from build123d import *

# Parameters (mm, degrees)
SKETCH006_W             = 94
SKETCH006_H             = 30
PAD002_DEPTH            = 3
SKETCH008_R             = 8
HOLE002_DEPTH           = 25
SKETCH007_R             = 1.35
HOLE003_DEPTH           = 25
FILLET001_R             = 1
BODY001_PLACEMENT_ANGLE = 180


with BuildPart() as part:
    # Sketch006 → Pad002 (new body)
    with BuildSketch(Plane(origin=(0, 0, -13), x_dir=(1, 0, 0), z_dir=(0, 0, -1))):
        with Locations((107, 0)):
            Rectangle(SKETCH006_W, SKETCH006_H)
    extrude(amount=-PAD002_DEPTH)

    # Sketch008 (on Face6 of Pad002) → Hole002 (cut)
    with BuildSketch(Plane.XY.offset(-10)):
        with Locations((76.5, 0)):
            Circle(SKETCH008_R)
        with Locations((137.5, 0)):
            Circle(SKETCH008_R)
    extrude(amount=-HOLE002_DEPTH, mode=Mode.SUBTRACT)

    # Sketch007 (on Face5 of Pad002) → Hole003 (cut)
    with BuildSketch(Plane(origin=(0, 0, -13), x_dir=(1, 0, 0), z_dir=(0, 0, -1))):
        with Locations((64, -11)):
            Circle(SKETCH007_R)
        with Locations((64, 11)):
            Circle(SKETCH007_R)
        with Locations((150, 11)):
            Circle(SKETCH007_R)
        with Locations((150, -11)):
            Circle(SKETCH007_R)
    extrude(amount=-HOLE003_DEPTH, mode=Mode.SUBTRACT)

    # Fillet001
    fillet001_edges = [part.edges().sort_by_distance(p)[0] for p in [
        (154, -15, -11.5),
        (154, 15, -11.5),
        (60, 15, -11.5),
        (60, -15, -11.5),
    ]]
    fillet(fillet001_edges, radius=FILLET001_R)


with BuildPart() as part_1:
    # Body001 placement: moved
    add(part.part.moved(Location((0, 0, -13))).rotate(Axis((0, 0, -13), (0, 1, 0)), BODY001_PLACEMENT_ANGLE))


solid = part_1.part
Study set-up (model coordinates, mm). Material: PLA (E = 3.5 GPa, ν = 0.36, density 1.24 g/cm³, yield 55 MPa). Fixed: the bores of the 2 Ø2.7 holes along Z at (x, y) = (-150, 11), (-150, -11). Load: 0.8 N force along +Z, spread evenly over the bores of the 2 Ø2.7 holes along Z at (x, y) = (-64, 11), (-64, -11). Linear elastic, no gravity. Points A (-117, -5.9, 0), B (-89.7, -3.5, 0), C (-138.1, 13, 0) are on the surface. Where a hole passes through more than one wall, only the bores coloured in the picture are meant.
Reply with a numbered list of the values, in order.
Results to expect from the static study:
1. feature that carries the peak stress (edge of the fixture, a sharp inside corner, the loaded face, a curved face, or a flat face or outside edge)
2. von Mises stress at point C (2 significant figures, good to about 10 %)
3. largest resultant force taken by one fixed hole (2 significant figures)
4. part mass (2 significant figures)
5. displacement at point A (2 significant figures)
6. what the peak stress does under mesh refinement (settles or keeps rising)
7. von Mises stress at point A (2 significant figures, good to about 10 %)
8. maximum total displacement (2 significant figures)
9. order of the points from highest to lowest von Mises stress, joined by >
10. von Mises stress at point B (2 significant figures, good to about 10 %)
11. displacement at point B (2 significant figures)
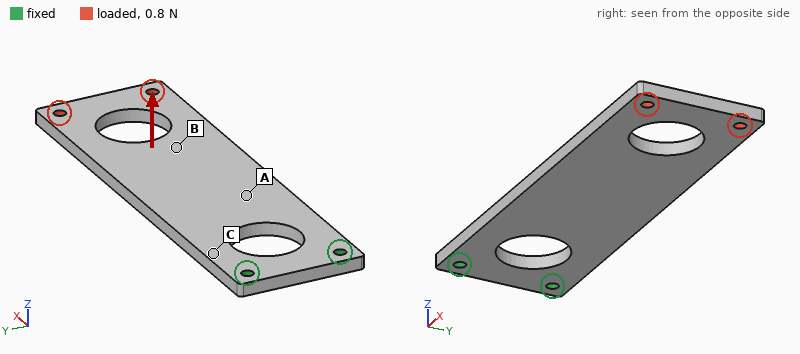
1. edge of the fixture
2. 2.6 MPa
3. 0.40 N
4. 8.9 g
5. 0.23 mm
6. keeps rising
7. 0.93 MPa
8. 1.1 mm
9. C > A > B
10. 0.41 MPa
11. 0.61 mm
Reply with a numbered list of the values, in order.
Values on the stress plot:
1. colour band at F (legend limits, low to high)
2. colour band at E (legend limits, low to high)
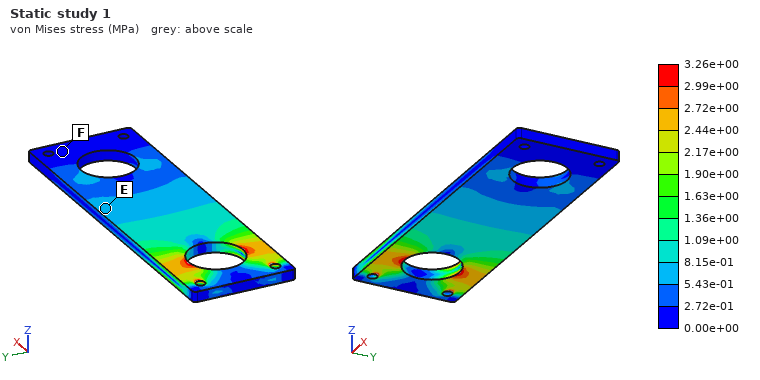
1. 0.00e+00 to 2.72e-01 MPa
2. 5.43e-01 to 8.15e-01 MPa
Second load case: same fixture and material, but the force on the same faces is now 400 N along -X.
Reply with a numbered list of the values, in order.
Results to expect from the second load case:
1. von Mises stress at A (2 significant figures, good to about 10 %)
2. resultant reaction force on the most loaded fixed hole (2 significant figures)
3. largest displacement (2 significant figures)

1. 3.9 MPa
2. 200 N
3. 0.19 mm
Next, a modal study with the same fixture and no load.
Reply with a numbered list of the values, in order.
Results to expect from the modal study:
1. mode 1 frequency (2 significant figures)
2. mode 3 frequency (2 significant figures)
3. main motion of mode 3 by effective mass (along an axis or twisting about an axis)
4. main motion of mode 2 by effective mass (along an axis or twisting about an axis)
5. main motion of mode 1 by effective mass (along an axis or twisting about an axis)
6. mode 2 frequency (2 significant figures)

1. 91 Hz
2. 590 Hz
3. along Z
4. twisting about X
5. along Z
6. 560 Hz
